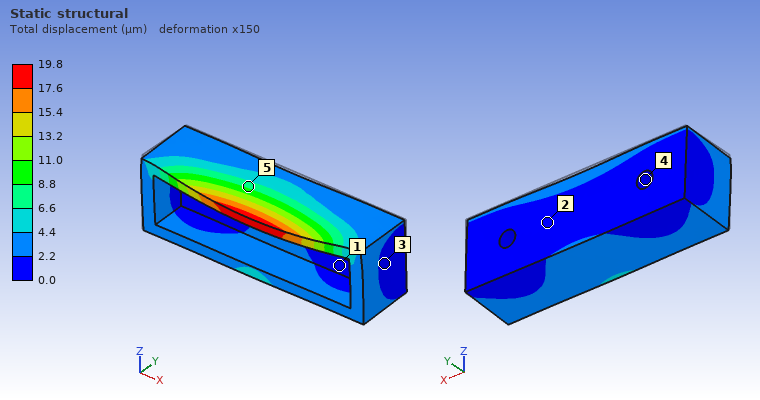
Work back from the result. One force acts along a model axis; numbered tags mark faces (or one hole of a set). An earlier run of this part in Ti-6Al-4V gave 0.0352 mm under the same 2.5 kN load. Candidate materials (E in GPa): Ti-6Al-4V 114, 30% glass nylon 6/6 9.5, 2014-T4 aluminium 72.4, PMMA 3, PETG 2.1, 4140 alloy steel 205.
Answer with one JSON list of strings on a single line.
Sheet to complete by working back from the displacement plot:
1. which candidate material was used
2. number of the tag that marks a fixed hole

["4140 alloy steel", "4"]
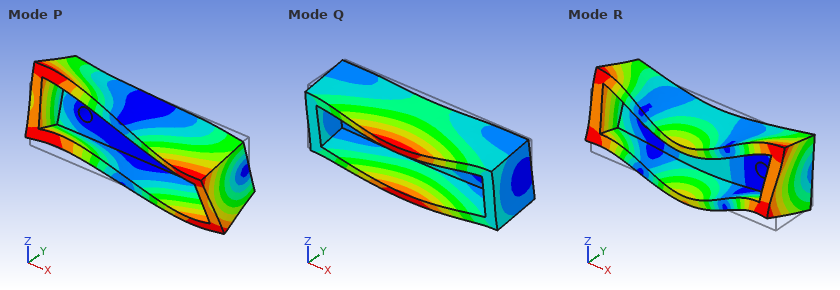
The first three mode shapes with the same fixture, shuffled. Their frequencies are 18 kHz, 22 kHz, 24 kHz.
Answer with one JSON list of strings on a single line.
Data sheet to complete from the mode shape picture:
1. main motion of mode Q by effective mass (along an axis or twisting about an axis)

["along Z"]
